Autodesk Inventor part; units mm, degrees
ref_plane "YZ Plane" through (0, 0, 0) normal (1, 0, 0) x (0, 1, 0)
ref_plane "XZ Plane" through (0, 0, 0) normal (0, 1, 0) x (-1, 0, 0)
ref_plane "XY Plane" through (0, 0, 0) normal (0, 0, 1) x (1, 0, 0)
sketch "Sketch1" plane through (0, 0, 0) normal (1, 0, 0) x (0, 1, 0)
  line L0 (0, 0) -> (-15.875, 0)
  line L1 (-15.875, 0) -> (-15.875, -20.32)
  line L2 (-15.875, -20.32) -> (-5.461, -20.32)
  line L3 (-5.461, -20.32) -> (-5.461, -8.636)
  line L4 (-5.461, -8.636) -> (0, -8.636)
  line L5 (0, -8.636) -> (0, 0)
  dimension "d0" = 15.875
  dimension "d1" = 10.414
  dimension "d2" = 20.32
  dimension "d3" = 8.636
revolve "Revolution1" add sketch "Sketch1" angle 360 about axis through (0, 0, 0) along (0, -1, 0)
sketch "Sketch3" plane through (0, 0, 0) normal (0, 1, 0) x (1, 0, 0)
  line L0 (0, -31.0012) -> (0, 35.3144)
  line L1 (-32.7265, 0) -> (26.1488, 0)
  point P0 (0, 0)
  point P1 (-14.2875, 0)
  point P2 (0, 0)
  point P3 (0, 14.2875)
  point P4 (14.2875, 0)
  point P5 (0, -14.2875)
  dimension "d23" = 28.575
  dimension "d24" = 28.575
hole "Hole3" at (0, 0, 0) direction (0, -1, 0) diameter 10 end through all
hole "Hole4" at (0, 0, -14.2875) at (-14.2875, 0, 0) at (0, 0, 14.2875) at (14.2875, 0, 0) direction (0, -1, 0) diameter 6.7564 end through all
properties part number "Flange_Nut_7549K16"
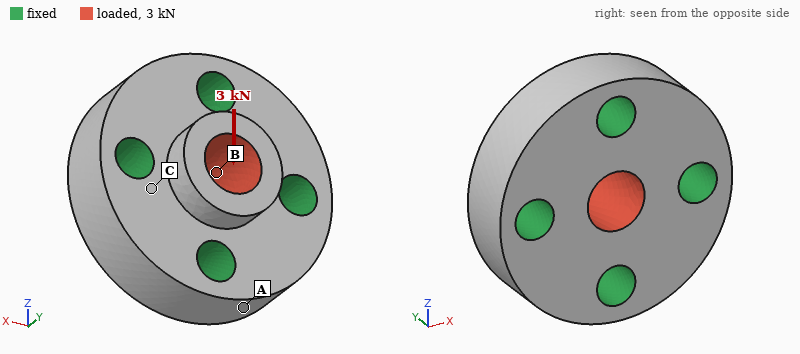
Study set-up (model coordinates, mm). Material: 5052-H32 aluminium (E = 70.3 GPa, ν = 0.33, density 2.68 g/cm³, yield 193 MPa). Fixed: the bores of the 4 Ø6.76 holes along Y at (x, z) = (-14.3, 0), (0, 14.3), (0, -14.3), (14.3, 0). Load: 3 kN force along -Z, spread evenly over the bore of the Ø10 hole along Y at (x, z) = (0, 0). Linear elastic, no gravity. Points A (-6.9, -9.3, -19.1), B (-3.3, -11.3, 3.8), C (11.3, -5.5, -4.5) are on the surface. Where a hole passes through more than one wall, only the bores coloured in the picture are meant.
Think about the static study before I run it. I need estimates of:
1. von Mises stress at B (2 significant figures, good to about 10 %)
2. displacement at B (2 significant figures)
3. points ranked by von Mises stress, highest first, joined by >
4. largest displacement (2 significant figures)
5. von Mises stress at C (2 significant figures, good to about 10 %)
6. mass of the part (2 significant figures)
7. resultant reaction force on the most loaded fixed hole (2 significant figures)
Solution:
8.6 MPa
0.84 µm
B > C > A
3.5 µm
4.4 MPa
32 g
1.0 kN
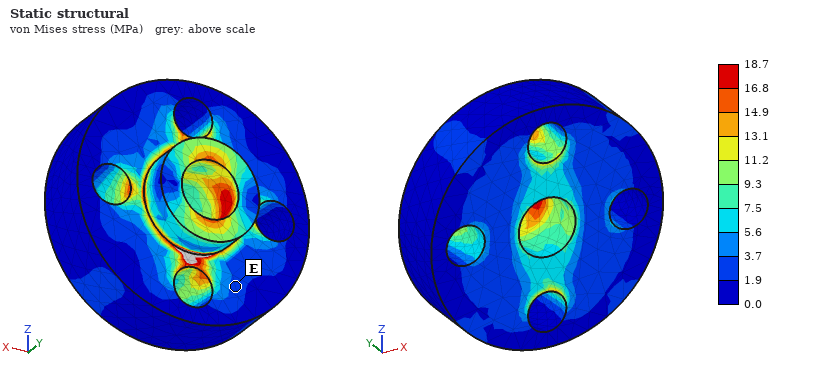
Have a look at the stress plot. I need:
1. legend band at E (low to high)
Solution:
1.9 to 3.7 MPa
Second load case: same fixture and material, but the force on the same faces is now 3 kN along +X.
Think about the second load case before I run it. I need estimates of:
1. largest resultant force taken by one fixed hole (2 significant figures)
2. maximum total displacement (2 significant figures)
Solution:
1.0 kN
3.5 µm
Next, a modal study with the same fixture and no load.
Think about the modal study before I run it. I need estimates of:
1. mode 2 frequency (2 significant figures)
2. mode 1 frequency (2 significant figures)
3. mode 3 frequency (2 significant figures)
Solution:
63 kHz
62 kHz
63 kHz
